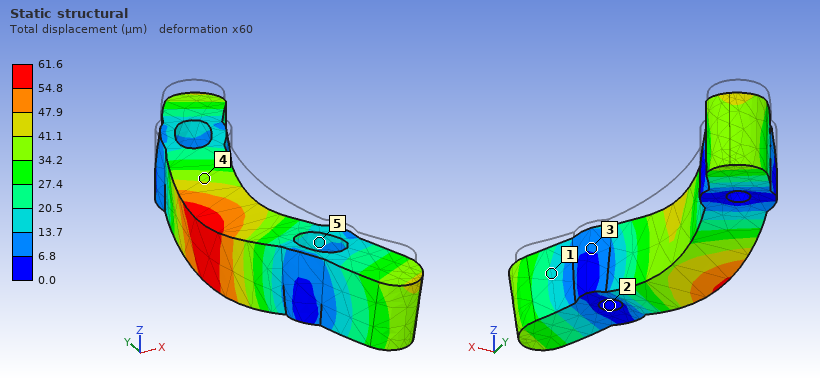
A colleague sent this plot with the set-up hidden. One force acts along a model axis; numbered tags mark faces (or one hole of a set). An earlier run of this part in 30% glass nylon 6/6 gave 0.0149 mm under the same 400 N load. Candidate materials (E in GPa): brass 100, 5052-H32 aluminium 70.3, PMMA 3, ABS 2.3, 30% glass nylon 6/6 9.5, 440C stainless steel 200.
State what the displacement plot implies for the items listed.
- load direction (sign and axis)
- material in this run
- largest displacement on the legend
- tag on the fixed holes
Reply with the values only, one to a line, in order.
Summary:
-Z
ABS
61.6 µm
2
